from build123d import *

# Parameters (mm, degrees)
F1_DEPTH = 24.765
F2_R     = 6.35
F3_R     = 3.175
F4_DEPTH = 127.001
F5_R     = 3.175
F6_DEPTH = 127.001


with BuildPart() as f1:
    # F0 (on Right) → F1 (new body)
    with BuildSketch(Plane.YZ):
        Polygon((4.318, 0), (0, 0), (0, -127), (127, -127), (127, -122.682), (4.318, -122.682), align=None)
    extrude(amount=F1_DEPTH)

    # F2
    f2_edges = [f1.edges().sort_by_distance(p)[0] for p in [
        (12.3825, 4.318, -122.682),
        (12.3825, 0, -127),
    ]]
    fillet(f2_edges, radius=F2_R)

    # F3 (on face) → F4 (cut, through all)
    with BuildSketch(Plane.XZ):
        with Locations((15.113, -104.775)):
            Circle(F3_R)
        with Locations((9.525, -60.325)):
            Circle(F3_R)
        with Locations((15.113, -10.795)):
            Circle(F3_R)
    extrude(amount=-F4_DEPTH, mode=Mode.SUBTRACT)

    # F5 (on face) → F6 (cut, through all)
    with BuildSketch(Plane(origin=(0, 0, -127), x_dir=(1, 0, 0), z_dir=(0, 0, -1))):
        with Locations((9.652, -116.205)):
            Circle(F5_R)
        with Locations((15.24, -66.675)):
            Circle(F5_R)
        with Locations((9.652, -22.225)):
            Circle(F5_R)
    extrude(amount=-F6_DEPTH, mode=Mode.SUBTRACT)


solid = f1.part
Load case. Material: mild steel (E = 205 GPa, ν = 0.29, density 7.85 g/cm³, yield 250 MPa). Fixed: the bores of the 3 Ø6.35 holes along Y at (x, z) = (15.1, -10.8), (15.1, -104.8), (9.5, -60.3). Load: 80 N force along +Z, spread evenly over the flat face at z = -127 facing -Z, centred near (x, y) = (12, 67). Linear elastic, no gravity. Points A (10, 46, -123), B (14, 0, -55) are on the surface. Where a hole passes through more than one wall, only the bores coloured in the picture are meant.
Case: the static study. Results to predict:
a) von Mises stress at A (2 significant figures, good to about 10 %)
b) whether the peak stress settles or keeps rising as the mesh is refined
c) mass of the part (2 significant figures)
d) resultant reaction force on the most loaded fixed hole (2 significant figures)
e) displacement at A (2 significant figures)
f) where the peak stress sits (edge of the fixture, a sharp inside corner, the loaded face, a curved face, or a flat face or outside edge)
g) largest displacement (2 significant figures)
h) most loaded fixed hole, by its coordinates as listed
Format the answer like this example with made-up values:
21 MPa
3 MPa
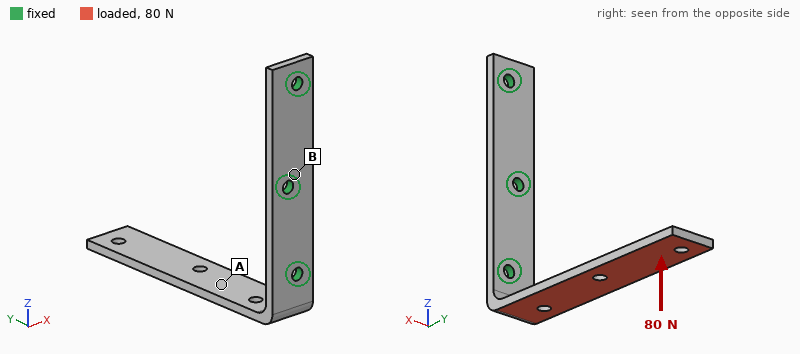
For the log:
28 MPa
keeps rising
200 g
74 N
0.19 mm
edge of the fixture
0.83 mm
(15.1, -104.8)
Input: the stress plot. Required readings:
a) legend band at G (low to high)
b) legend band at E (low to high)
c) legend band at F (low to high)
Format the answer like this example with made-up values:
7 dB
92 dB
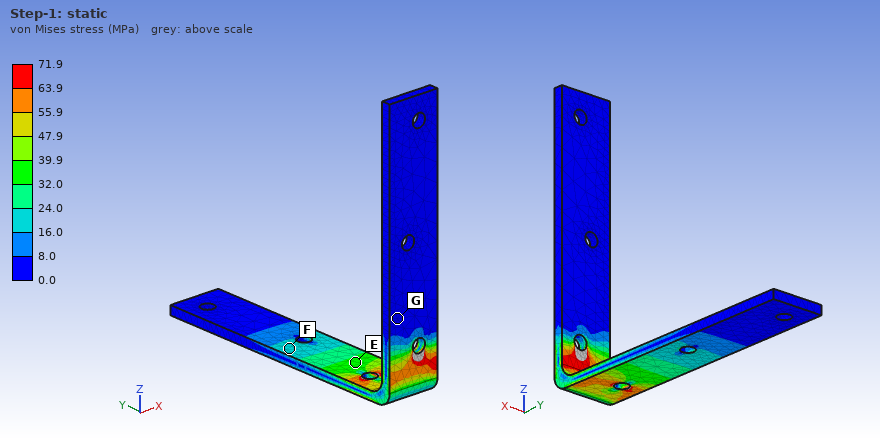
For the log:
0.0 to 8.0 MPa
32.0 to 39.9 MPa
16.0 to 24.0 MPa
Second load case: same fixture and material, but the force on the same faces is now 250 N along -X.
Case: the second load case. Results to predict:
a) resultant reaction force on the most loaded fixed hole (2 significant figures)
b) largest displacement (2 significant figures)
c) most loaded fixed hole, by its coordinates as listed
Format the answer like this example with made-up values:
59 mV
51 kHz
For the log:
330 N
0.58 mm
(15.1, -104.8)
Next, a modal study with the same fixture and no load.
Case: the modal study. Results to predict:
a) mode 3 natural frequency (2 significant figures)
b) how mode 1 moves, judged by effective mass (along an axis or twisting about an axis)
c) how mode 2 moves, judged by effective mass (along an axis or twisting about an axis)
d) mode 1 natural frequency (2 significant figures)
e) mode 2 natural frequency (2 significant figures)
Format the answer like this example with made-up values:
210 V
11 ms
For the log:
1200 Hz
along Z
along X
200 Hz
410 Hz
